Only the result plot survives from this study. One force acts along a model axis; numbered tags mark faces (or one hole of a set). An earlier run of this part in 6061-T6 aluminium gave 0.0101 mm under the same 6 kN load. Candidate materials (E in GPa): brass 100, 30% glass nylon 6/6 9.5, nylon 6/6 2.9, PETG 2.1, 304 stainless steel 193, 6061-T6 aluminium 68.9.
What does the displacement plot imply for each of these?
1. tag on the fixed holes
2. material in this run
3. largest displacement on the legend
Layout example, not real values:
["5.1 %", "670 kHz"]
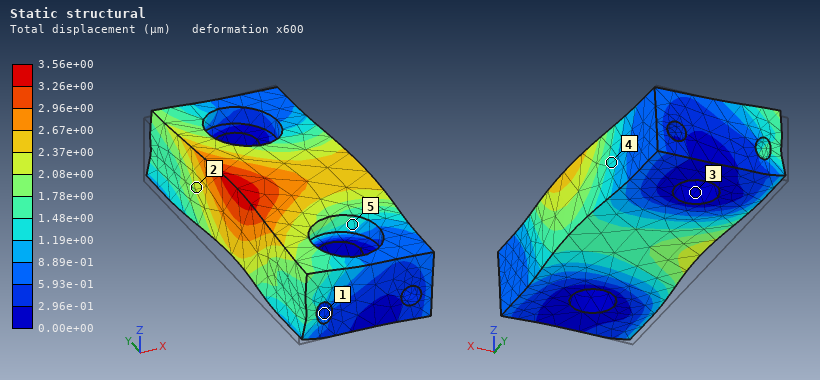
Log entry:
["3", "304 stainless steel", "3.56e+00 µm"]
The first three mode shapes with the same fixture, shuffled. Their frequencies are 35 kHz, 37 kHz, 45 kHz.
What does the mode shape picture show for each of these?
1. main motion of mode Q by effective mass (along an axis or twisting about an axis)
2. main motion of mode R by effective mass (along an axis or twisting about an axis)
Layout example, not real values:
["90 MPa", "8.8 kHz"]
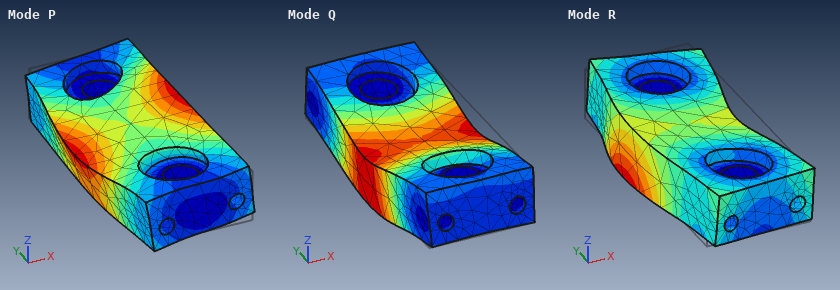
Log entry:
["along Z", "along X"]
